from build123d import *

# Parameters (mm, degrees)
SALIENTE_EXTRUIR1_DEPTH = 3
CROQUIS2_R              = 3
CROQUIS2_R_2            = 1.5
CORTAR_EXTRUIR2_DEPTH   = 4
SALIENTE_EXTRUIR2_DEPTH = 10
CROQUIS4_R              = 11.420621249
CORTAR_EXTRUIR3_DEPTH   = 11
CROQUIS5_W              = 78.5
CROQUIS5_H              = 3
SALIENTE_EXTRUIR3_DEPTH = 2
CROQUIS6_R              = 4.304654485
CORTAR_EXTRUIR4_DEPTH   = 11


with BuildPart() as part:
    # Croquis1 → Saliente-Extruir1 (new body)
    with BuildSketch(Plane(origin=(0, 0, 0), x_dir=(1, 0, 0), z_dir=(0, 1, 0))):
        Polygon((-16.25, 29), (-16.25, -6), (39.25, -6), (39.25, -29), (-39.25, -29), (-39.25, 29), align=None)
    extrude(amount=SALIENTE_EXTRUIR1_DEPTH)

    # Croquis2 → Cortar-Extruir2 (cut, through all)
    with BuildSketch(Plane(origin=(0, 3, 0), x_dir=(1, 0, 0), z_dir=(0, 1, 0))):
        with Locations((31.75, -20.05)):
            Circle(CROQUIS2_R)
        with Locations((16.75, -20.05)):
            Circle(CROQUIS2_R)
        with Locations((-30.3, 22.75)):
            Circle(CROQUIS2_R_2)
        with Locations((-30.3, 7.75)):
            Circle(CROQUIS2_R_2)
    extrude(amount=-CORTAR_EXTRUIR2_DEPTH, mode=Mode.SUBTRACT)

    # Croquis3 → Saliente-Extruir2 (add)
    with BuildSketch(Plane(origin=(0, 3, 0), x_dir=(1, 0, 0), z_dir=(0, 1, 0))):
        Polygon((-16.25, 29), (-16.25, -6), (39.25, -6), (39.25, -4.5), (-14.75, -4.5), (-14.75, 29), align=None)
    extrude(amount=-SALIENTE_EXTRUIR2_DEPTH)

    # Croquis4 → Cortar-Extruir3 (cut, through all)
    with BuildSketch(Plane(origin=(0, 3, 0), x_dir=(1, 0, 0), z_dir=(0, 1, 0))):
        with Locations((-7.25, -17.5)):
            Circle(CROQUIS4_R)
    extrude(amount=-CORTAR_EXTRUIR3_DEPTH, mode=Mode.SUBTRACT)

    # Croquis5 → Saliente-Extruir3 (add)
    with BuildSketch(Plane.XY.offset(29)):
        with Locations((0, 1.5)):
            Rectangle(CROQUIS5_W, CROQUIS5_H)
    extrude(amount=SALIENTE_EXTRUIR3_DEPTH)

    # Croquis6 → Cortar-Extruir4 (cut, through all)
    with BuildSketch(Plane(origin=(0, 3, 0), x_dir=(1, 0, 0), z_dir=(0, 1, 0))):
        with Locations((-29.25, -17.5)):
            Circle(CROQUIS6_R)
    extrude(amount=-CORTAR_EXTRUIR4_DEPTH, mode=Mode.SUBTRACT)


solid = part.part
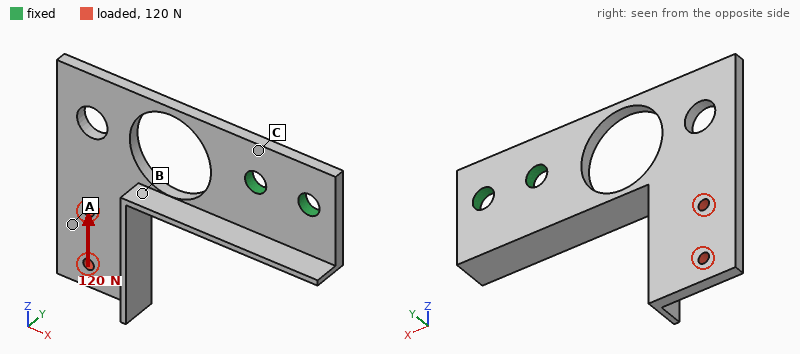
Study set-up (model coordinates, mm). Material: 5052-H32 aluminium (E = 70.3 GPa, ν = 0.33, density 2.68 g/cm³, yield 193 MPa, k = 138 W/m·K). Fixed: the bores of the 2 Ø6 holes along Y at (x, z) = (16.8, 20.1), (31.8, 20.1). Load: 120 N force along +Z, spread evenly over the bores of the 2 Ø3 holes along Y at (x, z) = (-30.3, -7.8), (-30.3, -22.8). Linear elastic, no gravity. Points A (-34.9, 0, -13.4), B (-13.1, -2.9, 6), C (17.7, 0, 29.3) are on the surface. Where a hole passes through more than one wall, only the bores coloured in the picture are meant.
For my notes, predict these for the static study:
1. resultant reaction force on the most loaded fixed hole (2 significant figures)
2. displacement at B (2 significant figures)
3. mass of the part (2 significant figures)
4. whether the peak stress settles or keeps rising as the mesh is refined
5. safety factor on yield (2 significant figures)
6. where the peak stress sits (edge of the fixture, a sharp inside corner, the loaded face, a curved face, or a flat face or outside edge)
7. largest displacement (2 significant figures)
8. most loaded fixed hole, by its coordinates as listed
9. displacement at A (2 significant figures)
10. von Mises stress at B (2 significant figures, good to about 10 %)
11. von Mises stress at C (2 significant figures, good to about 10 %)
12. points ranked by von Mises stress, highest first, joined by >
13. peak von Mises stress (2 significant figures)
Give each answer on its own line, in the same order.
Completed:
340 N
0.067 mm
21 g
settles
2.2
a curved face
0.11 mm
(16.8, 20.1)
0.10 mm
24 MPa
12 MPa
B > C > A
87 MPa
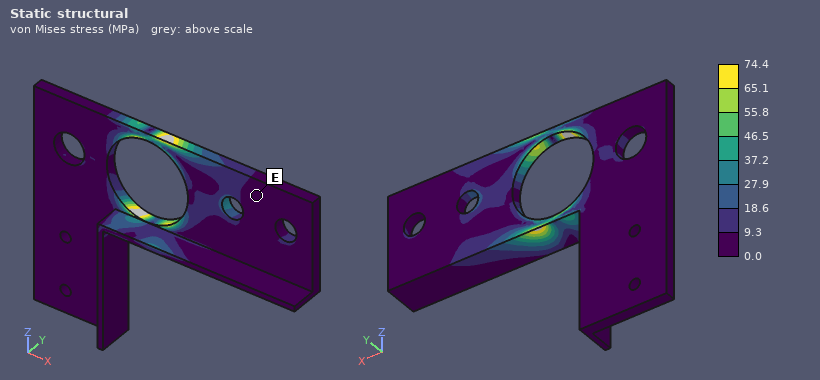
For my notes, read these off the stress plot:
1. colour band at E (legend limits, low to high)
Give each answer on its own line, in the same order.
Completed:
0.0 to 9.3 MPa
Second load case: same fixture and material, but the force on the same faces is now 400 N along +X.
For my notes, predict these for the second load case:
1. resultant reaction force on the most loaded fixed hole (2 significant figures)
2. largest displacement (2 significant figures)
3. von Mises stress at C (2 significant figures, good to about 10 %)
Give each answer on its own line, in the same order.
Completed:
620 N
0.34 mm
23 MPa
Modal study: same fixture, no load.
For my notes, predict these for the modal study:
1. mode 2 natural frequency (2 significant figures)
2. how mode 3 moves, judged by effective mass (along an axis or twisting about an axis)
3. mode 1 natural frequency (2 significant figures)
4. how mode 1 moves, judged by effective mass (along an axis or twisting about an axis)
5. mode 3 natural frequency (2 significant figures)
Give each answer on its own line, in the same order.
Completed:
980 Hz
along Z
540 Hz
along Y
1800 Hz
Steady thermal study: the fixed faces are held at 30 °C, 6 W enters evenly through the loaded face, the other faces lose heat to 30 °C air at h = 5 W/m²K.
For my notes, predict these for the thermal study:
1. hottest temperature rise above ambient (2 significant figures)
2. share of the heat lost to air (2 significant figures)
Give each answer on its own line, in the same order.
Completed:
53 K
15 %
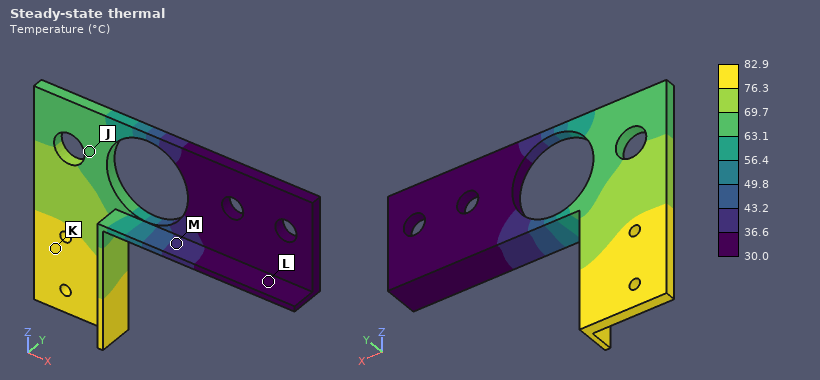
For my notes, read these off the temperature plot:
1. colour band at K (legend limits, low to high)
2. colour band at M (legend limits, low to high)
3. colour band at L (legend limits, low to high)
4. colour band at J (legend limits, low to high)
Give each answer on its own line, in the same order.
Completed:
76.3 to 82.9 °C
36.6 to 43.2 °C
30.0 to 36.6 °C
63.1 to 69.7 °C
